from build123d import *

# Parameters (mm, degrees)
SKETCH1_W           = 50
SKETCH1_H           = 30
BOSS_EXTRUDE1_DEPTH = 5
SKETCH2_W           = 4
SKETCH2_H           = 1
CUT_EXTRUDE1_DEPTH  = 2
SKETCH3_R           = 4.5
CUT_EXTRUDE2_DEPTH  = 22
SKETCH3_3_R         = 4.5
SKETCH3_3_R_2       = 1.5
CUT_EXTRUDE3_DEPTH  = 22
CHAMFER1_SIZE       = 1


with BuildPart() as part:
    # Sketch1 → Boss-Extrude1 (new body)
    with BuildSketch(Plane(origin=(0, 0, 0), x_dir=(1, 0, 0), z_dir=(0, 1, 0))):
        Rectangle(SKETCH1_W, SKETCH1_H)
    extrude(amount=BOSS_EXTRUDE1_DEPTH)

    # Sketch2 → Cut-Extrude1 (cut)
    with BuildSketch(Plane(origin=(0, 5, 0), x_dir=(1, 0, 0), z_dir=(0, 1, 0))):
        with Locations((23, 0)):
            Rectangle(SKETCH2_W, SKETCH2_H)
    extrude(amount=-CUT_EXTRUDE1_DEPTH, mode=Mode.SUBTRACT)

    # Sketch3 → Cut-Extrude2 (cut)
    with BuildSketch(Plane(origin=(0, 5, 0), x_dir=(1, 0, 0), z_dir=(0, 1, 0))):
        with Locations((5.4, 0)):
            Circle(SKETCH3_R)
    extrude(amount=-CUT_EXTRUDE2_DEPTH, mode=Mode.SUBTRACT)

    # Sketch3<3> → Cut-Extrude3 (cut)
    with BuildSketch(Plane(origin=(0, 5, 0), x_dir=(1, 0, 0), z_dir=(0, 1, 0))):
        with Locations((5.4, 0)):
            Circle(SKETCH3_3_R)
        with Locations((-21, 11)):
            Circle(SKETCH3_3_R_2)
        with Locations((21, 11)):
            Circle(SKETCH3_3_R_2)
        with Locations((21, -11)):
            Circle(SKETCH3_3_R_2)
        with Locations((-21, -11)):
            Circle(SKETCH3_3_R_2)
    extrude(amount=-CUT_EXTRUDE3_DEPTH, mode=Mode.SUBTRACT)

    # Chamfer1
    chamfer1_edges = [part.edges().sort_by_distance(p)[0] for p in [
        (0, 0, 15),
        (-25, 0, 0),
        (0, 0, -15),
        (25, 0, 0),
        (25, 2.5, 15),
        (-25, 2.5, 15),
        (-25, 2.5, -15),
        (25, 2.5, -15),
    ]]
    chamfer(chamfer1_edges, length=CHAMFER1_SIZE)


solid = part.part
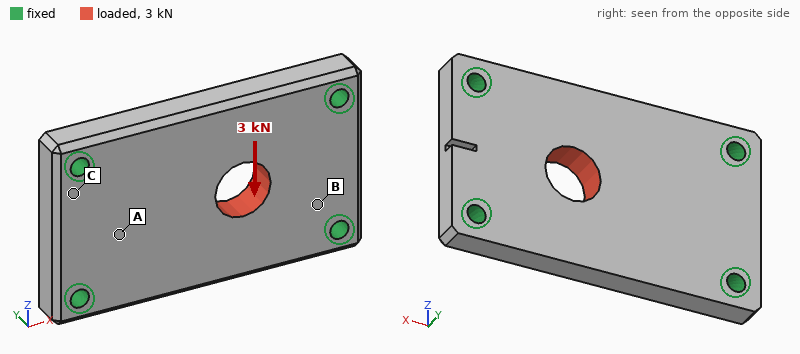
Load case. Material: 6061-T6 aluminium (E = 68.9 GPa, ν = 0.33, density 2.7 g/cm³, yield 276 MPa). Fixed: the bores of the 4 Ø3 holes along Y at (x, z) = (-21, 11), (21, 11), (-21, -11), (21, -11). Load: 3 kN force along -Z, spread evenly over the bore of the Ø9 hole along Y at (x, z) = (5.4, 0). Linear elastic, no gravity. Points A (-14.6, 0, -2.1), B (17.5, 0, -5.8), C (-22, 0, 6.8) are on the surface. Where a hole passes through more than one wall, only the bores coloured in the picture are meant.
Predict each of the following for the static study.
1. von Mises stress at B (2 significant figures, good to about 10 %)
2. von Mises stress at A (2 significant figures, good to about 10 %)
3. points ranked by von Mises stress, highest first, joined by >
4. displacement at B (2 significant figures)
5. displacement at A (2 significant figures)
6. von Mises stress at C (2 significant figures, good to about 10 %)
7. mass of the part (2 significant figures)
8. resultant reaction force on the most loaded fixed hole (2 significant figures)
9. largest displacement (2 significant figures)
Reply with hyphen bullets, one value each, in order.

- 27 MPa
- 16 MPa
- B > A > C
- 2.5 µm
- 2.8 µm
- 7.4 MPa
- 19 g
- 1.1 kN
- 11 µm
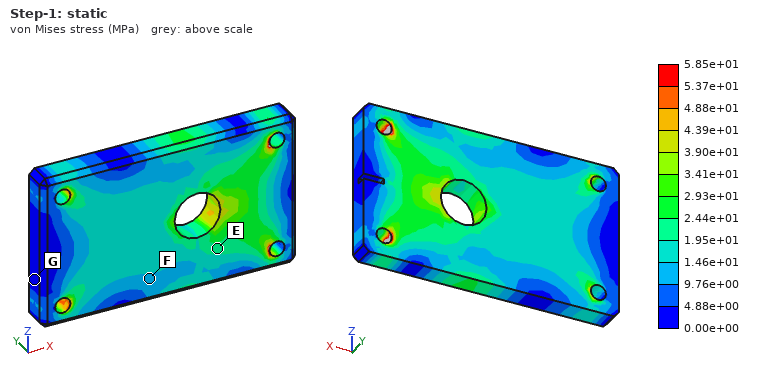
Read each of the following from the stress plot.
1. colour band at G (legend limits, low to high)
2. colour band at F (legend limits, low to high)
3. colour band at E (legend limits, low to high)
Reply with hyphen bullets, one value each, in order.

- 0.00e+00 to 4.88e+00 MPa
- 9.76e+00 to 1.46e+01 MPa
- 1.95e+01 to 2.44e+01 MPa
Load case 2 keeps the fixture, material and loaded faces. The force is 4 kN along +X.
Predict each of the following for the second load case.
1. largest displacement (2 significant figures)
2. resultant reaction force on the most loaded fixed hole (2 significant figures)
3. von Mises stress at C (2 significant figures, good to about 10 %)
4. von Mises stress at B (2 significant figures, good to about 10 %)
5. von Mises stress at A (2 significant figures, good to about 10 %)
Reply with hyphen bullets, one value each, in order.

- 6.8 µm
- 1.2 kN
- 8.8 MPa
- 25 MPa
- 7.9 MPa
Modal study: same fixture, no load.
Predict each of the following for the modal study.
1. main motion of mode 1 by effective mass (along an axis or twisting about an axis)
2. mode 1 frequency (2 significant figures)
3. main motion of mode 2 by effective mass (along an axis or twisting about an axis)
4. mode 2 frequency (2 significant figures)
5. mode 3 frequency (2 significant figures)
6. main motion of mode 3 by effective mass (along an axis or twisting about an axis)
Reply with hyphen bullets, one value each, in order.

- along Y
- 12 kHz
- twisting about X
- 18 kHz
- 30 kHz
- twisting about Z
